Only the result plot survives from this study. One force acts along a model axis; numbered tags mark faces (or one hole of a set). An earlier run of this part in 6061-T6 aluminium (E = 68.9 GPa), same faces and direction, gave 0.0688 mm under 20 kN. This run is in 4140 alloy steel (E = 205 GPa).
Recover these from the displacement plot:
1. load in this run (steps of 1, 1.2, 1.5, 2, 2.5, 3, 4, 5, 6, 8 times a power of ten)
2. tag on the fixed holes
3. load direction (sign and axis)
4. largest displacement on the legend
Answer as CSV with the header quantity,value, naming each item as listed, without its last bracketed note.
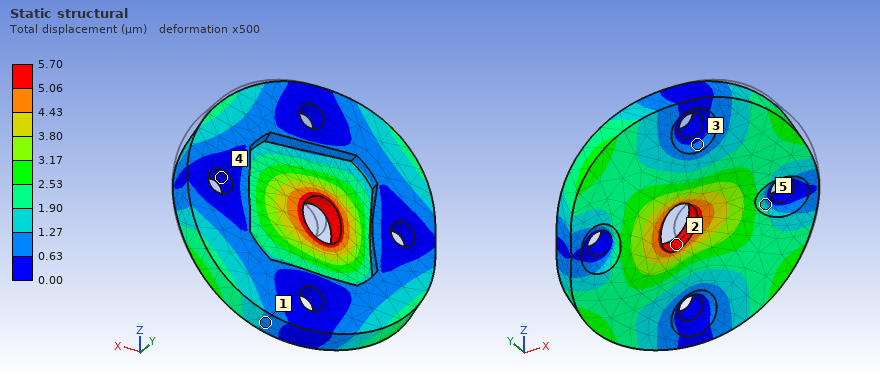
quantity,value
load in this run,5 kN
tag on the fixed holes,4
load direction,-X
largest displacement on the legend,5.70 µm
